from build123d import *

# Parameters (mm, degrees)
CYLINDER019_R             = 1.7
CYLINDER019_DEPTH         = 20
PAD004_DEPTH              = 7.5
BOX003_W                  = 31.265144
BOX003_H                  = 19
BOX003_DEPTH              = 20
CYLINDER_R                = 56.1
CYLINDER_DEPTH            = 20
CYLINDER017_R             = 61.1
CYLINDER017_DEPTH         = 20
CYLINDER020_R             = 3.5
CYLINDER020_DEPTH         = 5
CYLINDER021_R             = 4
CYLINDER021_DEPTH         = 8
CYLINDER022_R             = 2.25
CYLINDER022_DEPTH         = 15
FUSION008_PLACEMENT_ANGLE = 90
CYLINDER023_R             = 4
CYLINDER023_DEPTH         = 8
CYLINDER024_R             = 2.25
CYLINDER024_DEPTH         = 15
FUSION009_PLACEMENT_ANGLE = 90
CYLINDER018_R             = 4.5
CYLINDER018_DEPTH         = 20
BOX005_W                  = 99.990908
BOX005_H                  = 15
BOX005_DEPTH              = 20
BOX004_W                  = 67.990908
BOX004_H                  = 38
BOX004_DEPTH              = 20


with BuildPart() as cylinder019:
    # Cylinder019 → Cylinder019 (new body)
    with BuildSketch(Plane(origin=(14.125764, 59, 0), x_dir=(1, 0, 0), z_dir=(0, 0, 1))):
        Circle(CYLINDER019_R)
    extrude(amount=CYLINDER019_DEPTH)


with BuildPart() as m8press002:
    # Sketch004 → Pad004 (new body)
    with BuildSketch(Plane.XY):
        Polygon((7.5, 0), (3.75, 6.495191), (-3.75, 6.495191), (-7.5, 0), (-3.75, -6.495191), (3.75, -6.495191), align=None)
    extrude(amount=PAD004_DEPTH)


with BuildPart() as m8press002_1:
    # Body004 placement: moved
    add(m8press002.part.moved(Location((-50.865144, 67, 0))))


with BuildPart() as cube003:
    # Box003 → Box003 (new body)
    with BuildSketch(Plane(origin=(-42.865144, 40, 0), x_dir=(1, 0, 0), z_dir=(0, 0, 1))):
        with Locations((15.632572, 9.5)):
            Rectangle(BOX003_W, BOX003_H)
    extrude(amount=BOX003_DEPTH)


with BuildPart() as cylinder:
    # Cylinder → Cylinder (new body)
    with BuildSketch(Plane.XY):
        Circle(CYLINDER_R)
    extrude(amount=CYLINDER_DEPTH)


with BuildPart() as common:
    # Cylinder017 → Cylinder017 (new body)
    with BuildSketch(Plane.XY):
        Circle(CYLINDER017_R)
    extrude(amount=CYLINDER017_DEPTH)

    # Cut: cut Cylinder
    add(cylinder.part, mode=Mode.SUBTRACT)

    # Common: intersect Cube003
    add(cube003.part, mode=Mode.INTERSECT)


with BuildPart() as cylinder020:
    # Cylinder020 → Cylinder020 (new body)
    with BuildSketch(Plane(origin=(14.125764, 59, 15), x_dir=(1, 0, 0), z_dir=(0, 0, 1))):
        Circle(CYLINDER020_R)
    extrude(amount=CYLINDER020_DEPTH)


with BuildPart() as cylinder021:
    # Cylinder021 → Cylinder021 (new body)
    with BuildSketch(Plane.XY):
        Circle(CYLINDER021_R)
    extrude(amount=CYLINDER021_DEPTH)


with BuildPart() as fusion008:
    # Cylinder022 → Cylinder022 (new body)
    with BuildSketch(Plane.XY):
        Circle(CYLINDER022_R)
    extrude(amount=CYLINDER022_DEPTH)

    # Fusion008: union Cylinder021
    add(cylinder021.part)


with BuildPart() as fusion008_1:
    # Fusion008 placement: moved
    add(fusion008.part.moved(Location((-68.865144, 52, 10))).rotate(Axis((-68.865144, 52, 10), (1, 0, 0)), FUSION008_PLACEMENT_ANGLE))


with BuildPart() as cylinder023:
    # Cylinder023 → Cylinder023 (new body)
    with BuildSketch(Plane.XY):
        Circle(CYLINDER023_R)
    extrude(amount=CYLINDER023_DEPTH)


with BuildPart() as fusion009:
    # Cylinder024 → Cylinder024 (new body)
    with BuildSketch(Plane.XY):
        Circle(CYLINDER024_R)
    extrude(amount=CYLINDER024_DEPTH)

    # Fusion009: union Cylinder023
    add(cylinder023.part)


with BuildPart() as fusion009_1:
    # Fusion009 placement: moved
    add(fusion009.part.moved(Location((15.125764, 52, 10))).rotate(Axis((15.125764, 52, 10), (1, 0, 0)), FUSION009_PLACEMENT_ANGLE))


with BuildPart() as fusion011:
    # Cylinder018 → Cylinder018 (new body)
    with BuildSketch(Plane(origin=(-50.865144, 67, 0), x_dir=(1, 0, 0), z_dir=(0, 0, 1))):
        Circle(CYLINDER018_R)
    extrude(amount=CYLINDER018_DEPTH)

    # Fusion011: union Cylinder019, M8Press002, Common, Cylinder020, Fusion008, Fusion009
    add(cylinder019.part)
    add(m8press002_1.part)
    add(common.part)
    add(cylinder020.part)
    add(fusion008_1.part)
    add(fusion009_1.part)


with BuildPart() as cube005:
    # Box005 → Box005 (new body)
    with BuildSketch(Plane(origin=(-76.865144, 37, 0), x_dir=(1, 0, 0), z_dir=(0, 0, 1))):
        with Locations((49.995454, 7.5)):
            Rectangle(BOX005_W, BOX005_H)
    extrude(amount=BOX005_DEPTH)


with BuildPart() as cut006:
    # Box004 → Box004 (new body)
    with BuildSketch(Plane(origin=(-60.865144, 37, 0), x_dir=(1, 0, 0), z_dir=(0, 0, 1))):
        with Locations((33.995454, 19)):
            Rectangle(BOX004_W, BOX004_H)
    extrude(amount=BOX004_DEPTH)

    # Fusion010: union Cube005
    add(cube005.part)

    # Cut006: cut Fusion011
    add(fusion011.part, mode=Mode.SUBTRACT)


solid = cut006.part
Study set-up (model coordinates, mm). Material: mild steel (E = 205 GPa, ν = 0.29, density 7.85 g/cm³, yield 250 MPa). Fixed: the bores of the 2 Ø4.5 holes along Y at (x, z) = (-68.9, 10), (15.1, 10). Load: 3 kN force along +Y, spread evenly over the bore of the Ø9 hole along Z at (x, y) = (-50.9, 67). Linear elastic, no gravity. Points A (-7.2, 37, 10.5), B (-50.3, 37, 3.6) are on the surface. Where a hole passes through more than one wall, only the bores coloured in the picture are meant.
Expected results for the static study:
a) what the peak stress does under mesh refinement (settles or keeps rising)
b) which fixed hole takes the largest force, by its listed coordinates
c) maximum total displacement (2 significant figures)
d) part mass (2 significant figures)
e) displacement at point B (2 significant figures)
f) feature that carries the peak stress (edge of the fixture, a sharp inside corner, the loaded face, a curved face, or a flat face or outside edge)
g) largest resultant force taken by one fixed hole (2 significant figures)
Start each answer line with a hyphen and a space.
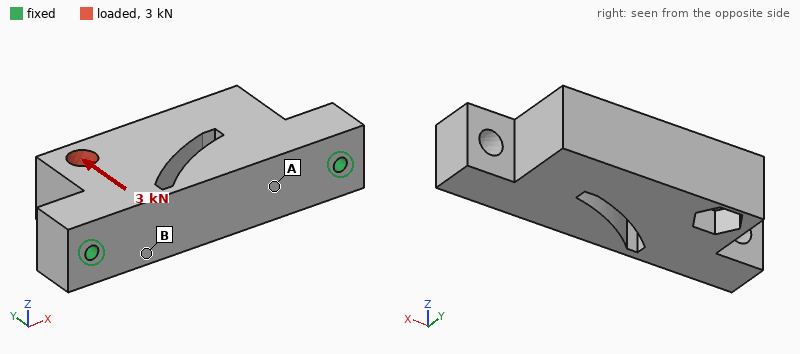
- keeps rising
- (-68.9, 10)
- 12 µm
- 430 g
- 2.6 µm
- edge of the fixture
- 2.5 kN
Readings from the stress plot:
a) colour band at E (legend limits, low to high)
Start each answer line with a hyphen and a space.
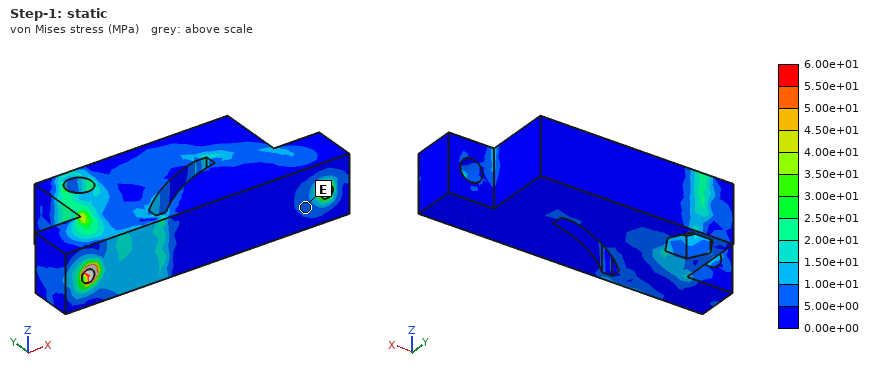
- 5.00e+00 to 1.00e+01 MPa
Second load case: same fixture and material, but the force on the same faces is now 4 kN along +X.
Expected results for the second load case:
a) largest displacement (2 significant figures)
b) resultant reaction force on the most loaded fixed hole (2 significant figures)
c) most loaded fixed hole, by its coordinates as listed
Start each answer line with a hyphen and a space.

- 6.4 µm
- 2.6 kN
- (-68.9, 10)
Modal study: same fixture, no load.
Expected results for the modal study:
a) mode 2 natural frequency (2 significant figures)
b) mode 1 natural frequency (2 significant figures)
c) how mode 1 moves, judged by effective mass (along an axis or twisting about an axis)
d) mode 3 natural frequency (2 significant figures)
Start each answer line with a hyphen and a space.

- 8400 Hz
- 2900 Hz
- along Z
- 8500 Hz
